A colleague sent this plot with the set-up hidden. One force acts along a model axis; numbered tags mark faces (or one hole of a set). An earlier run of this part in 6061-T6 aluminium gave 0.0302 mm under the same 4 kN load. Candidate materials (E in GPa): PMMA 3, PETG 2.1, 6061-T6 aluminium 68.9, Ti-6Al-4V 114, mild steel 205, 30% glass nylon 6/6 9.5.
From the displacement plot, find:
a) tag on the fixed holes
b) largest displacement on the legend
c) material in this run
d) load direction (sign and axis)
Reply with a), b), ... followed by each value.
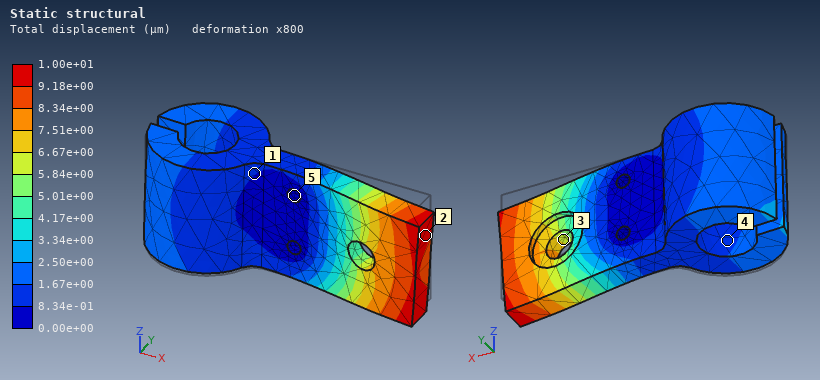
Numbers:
a) 5
b) 1.00e+01 µm
c) mild steel
d) -Z
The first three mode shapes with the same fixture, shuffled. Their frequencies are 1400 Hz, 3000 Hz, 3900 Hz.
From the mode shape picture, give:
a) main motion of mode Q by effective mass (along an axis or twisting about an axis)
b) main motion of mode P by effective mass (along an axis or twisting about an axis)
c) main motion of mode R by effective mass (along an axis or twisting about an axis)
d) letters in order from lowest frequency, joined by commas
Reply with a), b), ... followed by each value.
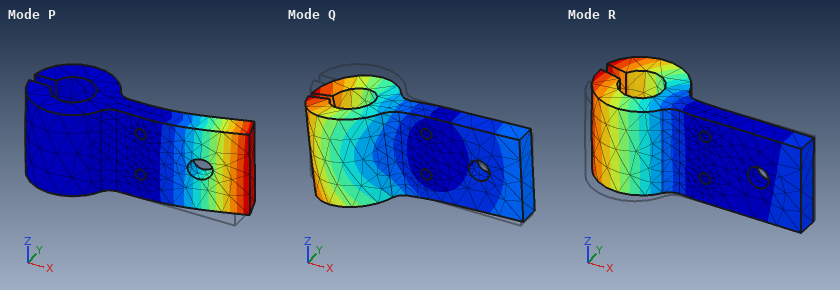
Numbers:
a) along Z
b) along Y
c) along Y
d) R, P, Q
